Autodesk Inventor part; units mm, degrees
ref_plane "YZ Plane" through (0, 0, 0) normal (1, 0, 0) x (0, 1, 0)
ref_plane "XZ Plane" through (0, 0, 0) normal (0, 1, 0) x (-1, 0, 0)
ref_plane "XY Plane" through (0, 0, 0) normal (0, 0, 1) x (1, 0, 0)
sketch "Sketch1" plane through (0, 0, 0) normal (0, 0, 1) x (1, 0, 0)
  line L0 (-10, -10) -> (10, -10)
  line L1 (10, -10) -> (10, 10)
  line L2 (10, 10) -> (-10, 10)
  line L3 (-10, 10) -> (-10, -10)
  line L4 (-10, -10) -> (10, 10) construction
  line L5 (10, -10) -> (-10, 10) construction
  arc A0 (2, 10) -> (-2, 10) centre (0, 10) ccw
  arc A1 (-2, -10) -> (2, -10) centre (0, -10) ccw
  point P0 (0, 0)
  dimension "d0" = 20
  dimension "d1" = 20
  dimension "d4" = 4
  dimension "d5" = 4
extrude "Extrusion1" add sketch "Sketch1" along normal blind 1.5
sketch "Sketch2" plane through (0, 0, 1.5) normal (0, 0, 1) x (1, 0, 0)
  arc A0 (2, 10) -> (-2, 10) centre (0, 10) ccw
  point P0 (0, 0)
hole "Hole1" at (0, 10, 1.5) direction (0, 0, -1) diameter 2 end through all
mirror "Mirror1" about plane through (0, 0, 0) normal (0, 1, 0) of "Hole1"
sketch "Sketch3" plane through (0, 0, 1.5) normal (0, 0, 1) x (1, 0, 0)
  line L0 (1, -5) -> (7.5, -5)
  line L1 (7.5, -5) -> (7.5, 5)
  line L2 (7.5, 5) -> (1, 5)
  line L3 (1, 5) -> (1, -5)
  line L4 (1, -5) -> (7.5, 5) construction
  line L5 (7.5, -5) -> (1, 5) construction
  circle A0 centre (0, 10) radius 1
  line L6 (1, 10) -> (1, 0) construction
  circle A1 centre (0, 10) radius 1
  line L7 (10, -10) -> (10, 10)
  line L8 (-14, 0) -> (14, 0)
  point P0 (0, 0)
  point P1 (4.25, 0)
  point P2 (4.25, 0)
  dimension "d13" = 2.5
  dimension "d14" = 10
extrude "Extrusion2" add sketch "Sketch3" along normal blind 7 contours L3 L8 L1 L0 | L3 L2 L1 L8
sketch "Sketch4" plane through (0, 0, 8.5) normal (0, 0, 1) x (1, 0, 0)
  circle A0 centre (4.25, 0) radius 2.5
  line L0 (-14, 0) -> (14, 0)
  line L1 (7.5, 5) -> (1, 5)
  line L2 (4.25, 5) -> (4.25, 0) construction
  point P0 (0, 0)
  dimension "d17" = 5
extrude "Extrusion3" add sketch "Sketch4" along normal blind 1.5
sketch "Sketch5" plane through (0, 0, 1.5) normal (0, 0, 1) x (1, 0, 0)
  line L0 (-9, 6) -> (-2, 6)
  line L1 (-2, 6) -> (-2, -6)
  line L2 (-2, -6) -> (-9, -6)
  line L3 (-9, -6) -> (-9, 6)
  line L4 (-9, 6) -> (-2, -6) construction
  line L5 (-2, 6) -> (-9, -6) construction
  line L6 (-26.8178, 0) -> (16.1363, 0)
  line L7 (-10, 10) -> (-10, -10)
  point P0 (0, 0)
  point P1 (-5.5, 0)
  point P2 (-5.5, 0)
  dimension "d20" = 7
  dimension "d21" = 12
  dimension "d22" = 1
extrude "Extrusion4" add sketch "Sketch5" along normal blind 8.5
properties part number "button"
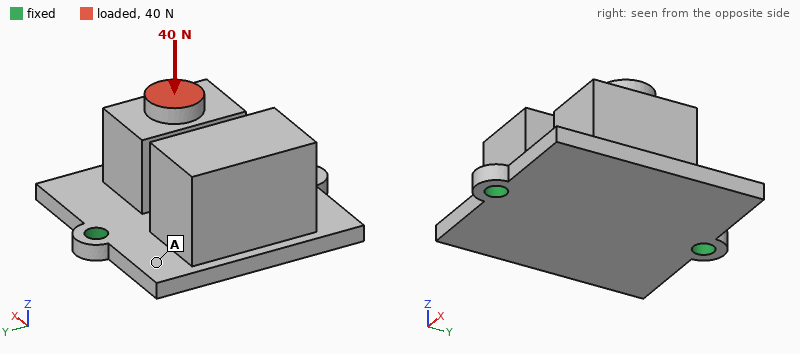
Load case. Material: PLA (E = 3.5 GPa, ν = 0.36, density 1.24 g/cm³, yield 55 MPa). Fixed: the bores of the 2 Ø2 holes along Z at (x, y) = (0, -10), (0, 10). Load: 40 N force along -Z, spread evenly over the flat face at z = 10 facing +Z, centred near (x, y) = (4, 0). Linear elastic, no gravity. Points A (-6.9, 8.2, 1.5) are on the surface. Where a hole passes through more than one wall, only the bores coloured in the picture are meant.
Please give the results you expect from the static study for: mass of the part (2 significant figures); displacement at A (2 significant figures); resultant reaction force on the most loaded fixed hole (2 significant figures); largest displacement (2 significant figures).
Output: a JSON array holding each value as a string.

["2.2 g", "0.087 mm", "21 N", "0.35 mm"]
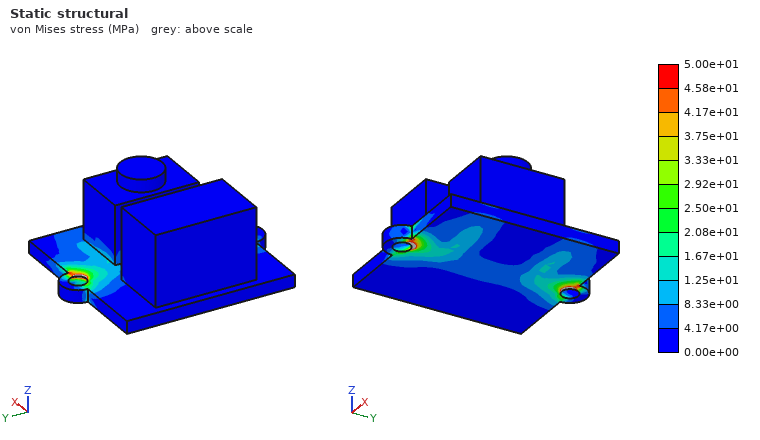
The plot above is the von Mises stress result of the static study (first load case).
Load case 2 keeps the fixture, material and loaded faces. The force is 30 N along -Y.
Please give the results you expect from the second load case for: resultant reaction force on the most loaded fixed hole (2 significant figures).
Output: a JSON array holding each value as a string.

["24 N"]
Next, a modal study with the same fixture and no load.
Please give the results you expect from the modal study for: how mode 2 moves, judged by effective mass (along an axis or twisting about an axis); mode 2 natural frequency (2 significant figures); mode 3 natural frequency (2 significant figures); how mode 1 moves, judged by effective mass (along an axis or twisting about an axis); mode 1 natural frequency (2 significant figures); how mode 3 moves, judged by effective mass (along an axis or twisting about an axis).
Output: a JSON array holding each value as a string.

["along Z", "2300 Hz", "4700 Hz", "along X", "1300 Hz", "along Z"]
